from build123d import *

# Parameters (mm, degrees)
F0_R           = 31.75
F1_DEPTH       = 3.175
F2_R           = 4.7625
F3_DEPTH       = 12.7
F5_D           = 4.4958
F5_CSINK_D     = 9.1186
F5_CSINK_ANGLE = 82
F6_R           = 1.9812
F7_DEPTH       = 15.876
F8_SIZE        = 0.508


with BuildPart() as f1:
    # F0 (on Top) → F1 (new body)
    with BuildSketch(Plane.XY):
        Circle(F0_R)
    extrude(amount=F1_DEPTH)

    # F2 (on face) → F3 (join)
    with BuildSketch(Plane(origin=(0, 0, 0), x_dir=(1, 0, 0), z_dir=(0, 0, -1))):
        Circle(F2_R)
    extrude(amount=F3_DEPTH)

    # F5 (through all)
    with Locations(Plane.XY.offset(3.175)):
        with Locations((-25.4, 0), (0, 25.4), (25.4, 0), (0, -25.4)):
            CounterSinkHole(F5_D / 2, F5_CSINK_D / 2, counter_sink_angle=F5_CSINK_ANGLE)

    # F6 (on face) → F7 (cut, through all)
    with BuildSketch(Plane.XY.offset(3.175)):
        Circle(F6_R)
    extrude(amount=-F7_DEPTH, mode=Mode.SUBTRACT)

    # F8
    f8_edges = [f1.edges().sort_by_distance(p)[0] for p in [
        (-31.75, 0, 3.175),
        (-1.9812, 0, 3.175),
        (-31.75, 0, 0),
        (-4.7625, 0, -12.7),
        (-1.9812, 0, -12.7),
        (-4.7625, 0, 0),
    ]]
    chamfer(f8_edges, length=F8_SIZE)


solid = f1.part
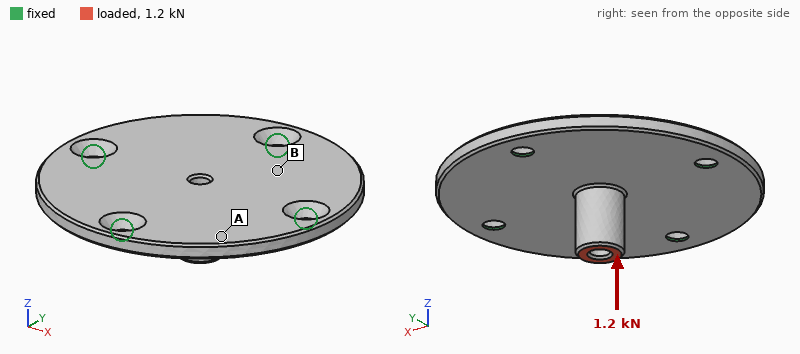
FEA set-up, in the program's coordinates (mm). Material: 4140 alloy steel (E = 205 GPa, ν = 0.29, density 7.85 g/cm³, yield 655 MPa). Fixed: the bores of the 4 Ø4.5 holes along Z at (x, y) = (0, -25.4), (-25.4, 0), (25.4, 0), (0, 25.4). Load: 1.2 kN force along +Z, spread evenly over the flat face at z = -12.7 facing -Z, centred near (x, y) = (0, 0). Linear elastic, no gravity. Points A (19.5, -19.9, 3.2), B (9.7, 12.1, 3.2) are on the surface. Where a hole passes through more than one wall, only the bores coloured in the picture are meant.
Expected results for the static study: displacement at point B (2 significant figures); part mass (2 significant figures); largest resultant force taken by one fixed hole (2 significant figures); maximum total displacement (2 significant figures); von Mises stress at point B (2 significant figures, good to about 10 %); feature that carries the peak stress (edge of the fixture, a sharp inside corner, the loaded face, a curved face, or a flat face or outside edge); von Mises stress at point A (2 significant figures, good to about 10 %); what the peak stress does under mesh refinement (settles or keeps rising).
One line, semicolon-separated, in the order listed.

16 µm; 81 g; 790 N; 34 µm; 53 MPa; edge of the fixture; 20 MPa; keeps rising
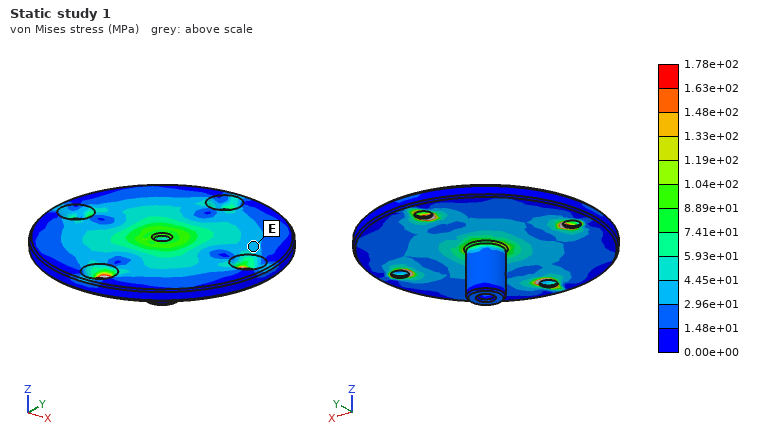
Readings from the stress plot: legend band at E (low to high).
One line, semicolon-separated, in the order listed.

2.96e+01 to 4.45e+01 MPa
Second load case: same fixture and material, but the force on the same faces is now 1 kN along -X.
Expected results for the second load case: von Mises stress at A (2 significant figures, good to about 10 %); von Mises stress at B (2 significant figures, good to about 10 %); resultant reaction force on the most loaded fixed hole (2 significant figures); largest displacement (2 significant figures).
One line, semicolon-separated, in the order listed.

21 MPa; 40 MPa; 520 N; 54 µm
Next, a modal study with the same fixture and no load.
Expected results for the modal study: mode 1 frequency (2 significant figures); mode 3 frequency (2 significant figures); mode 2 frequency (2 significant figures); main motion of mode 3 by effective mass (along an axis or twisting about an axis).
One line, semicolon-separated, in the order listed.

6900 Hz; 7900 Hz; 7200 Hz; twisting about X
